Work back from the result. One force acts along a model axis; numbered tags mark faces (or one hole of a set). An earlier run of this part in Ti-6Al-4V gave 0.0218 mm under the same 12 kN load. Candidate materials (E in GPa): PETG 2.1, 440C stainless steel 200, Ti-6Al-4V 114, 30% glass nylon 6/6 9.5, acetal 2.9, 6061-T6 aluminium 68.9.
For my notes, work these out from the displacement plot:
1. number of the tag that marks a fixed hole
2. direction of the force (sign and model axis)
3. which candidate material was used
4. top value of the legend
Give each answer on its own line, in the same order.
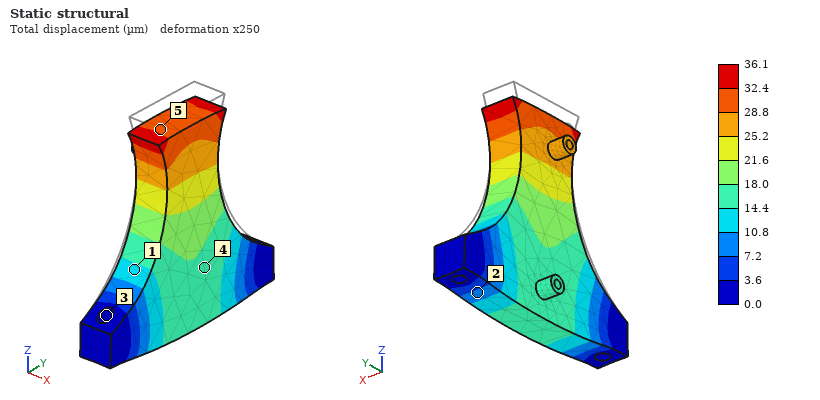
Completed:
3
-Z
6061-T6 aluminium
36.1 µm
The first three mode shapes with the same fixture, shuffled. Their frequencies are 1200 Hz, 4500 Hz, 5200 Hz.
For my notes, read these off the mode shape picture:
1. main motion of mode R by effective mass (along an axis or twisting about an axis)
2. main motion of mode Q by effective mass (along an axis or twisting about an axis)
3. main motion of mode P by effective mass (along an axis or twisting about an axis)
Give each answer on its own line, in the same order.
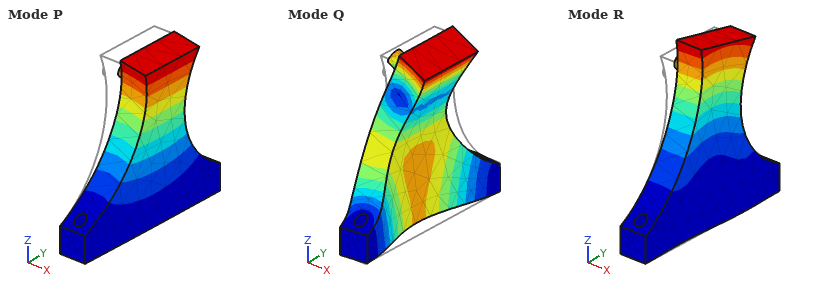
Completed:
along Y
along X
along X
